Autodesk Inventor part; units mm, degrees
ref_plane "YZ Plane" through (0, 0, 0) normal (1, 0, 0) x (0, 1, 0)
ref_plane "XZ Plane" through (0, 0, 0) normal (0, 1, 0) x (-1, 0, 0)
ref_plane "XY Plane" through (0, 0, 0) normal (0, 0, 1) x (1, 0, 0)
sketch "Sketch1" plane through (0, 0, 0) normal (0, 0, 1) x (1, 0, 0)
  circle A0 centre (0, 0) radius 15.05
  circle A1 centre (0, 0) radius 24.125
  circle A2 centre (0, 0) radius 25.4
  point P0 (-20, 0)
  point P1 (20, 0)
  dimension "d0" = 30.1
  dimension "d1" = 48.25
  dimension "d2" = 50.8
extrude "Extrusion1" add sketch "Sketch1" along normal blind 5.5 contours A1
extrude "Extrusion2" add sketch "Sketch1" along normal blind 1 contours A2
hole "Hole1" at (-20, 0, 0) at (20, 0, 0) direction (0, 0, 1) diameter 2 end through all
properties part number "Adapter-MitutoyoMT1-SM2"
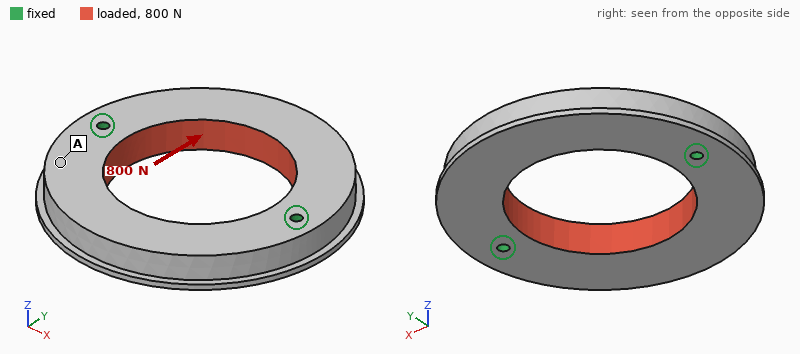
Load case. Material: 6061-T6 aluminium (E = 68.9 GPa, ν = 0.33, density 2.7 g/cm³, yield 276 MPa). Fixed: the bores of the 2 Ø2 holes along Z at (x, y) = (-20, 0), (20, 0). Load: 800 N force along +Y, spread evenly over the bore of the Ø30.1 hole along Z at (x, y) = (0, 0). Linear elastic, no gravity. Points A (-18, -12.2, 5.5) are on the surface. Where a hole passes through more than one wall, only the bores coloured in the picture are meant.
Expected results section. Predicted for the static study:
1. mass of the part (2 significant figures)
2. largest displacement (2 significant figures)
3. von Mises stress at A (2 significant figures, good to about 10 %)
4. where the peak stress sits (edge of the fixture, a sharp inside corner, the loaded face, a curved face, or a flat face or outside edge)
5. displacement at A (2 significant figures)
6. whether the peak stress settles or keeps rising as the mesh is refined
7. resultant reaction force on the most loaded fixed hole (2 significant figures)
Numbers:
17 g
2.3 µm
2.2 MPa
edge of the fixture
0.76 µm
keeps rising
400 N
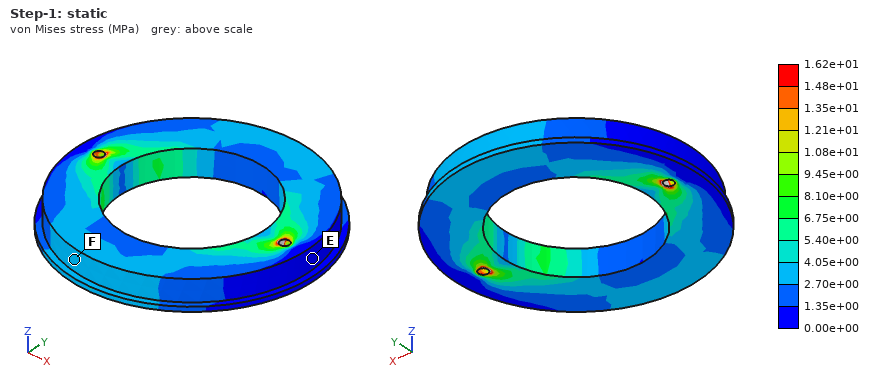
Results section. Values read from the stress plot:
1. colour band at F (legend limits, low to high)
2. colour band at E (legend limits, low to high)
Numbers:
2.70e+00 to 4.05e+00 MPa
0.00e+00 to 1.35e+00 MPa
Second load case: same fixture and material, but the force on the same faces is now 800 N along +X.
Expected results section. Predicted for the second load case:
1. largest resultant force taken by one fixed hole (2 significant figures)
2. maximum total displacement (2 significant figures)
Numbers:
400 N
4.2 µm
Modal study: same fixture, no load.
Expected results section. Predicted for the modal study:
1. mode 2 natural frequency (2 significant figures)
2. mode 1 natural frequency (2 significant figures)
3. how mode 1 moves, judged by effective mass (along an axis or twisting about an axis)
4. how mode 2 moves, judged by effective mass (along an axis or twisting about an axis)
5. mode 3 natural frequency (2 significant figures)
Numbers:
5800 Hz
5100 Hz
twisting about X
along Z
13 kHz
